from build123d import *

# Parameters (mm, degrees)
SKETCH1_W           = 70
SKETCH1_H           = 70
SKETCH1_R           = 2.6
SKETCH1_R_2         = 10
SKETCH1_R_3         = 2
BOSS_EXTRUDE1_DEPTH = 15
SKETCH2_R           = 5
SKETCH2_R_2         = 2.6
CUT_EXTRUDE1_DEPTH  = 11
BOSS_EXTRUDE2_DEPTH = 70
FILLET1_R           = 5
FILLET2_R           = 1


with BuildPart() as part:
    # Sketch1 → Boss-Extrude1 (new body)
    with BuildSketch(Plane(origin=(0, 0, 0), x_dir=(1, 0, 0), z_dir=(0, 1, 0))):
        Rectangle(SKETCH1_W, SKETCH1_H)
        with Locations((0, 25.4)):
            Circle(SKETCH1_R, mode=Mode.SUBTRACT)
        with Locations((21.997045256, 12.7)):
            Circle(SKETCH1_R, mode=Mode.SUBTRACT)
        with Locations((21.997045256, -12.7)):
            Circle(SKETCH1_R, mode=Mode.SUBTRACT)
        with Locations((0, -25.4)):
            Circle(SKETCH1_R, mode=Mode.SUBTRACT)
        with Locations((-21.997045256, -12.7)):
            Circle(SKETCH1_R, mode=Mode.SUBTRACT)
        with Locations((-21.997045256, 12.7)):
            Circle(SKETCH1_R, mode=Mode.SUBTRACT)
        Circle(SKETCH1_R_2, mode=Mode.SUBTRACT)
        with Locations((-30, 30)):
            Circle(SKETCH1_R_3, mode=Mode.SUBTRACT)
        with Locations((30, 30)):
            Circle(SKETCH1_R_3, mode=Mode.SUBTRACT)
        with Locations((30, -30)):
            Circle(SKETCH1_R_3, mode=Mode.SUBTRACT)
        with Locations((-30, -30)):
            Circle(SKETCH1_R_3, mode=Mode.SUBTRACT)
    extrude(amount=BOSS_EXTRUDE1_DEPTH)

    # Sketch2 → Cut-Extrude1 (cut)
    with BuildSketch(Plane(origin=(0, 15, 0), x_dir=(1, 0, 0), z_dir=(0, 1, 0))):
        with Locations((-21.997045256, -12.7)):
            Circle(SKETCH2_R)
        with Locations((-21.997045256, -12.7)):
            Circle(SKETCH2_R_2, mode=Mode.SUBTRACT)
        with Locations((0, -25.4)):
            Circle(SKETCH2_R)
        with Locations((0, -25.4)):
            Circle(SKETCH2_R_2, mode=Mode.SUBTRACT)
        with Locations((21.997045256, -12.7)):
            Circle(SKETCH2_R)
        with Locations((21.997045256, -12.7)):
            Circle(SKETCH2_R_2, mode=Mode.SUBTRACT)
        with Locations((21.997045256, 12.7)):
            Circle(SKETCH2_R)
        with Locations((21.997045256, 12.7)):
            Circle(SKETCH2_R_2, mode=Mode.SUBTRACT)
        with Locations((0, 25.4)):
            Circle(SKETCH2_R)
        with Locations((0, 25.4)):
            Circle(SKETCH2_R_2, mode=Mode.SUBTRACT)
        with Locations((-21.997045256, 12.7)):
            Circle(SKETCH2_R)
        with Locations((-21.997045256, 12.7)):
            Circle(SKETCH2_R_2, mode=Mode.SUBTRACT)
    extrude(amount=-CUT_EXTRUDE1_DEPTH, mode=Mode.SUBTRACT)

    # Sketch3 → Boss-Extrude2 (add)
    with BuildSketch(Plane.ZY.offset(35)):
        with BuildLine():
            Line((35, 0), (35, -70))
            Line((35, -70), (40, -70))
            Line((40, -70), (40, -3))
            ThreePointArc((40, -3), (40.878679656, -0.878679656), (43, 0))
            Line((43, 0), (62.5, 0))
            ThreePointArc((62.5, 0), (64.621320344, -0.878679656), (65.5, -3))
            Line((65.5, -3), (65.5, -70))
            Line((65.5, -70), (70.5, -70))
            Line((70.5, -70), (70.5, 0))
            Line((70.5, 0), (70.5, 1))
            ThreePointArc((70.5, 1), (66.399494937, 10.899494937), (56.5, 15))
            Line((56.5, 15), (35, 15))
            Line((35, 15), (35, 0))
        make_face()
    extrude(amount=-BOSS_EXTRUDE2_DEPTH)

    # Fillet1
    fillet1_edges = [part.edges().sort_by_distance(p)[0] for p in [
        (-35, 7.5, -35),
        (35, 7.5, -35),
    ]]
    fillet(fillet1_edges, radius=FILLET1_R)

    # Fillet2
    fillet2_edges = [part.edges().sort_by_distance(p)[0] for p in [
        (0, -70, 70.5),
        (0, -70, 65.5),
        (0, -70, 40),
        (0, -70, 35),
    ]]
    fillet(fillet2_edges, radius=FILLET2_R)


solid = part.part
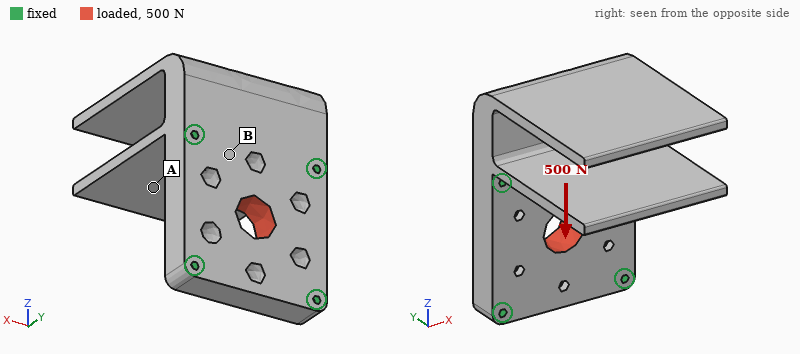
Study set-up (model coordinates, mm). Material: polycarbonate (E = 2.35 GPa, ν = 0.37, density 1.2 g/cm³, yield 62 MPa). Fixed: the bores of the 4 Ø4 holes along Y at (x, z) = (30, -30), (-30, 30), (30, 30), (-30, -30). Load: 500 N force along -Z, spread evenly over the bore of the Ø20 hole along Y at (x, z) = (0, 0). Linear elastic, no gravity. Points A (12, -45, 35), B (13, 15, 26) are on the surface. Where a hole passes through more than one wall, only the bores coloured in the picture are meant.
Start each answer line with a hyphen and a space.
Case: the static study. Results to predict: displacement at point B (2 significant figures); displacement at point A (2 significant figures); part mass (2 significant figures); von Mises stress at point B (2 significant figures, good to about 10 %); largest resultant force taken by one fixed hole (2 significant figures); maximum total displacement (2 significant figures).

- 5.3 µm
- 5.9 µm
- 170 g
- 0.35 MPa
- 150 N
- 13 µm
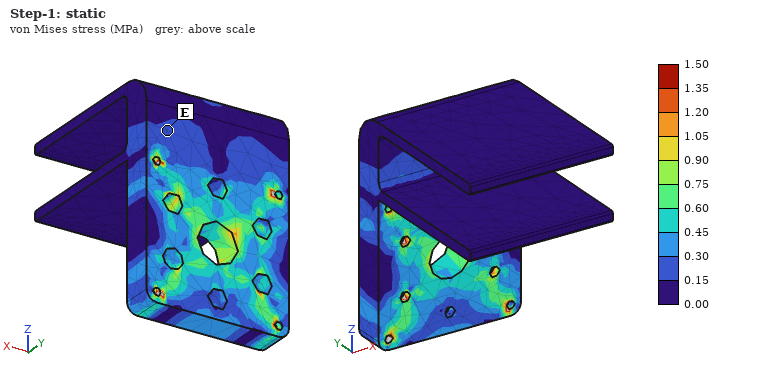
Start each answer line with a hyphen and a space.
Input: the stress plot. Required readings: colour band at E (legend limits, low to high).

- 0.15 to 0.30 MPa
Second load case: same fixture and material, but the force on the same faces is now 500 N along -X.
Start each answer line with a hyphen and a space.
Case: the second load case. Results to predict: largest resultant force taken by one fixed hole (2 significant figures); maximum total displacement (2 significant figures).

- 140 N
- 14 µm
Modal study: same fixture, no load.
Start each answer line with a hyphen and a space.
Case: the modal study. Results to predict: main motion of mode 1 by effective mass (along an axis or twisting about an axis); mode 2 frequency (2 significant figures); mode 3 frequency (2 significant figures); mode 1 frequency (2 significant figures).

- along Z
- 230 Hz
- 530 Hz
- 220 Hz
